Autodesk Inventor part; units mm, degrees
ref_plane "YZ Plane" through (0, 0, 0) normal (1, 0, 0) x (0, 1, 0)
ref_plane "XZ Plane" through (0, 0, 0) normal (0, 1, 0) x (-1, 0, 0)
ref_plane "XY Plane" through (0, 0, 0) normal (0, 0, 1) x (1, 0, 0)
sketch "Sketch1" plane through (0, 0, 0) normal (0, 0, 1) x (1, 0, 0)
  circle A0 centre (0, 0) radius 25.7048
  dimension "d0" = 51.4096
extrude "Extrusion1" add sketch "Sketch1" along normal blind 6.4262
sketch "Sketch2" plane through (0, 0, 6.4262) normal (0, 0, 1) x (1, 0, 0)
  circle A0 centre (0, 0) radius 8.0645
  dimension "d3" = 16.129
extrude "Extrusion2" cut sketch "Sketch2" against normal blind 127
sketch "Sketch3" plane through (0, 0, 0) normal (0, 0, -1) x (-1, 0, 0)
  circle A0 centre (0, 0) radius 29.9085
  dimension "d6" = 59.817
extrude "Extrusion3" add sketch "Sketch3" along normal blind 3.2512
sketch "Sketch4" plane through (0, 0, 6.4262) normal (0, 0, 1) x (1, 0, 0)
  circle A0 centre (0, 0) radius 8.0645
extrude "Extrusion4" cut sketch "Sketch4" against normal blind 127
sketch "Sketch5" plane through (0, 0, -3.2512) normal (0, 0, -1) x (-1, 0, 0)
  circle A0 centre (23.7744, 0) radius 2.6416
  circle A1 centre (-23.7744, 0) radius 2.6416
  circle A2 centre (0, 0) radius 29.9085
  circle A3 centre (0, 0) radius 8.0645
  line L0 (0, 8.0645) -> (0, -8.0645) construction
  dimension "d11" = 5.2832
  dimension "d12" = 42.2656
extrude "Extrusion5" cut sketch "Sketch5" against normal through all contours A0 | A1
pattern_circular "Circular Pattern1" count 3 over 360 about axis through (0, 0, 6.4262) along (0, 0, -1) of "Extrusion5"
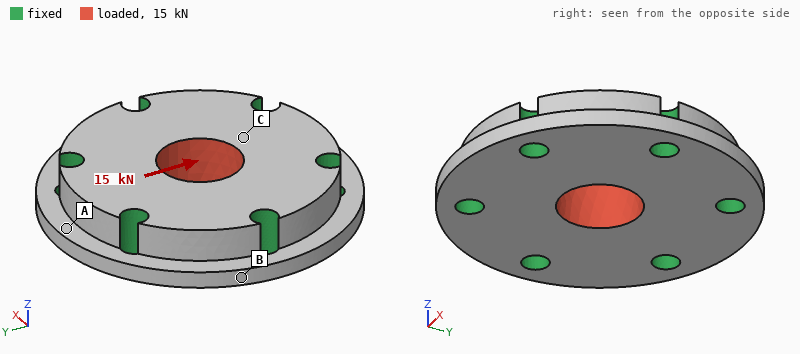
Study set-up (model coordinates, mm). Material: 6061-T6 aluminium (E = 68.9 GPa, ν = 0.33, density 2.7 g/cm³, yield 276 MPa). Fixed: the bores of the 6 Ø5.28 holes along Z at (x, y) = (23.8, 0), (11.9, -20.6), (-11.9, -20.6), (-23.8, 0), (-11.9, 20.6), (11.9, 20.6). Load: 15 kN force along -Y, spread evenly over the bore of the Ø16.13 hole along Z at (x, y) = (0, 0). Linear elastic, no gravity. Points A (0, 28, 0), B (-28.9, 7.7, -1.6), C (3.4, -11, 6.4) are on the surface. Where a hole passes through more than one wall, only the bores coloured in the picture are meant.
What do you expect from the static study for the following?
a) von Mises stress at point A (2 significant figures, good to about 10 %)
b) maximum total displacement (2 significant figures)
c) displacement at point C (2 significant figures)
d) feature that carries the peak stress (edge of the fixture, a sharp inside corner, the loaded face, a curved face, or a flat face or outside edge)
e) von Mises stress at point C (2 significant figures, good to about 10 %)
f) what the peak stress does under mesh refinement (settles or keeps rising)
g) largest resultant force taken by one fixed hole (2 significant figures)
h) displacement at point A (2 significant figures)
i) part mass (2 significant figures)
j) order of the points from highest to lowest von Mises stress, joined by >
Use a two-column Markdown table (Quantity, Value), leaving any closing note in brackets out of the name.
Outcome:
| Quantity | Value |
|---|---|
| von Mises stress at point A | 12 MPa |
| maximum total displacement | 7.5 µm |
| displacement at point C | 5.8 µm |
| feature that carries the peak stress | edge of the fixture |
| von Mises stress at point C | 28 MPa |
| what the peak stress does under mesh refinement | keeps rising |
| largest resultant force taken by one fixed hole | 3.4 kN |
| displacement at point A | 3.2 µm |
| part mass | 52 g |
| order of the points from highest to lowest von Mises stress, joined by > | C > A > B |
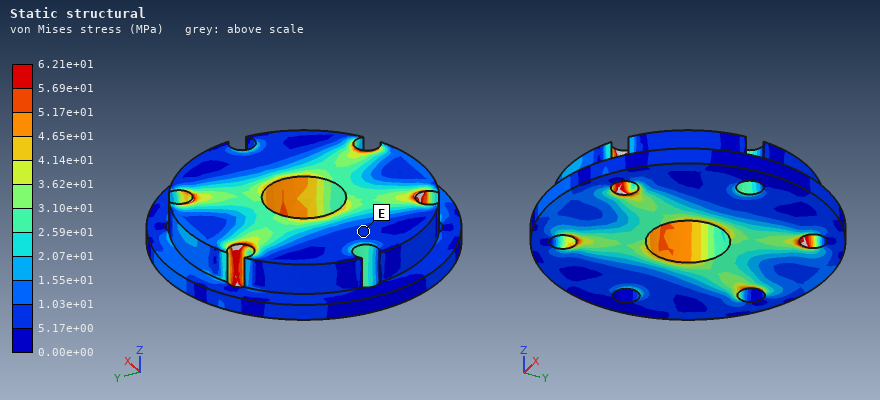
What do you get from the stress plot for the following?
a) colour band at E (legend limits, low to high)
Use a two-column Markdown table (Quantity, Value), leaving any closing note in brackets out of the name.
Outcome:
| Quantity | Value |
|---|---|
| colour band at E | 5.17e+00 to 1.03e+01 MPa |
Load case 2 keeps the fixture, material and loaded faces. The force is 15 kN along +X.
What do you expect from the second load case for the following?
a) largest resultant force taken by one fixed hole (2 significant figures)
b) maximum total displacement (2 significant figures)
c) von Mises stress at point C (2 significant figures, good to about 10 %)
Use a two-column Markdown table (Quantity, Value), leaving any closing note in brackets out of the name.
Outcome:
| Quantity | Value |
|---|---|
| largest resultant force taken by one fixed hole | 3.9 kN |
| maximum total displacement | 7.4 µm |
| von Mises stress at point C | 25 MPa |
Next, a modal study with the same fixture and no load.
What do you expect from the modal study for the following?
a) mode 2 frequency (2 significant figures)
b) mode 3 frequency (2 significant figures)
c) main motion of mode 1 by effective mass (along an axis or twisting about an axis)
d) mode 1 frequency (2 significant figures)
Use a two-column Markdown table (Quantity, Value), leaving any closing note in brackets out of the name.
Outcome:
| Quantity | Value |
|---|---|
| mode 2 frequency | 45 kHz |
| mode 3 frequency | 45 kHz |
| main motion of mode 1 by effective mass | along Z |
| mode 1 frequency | 32 kHz |
